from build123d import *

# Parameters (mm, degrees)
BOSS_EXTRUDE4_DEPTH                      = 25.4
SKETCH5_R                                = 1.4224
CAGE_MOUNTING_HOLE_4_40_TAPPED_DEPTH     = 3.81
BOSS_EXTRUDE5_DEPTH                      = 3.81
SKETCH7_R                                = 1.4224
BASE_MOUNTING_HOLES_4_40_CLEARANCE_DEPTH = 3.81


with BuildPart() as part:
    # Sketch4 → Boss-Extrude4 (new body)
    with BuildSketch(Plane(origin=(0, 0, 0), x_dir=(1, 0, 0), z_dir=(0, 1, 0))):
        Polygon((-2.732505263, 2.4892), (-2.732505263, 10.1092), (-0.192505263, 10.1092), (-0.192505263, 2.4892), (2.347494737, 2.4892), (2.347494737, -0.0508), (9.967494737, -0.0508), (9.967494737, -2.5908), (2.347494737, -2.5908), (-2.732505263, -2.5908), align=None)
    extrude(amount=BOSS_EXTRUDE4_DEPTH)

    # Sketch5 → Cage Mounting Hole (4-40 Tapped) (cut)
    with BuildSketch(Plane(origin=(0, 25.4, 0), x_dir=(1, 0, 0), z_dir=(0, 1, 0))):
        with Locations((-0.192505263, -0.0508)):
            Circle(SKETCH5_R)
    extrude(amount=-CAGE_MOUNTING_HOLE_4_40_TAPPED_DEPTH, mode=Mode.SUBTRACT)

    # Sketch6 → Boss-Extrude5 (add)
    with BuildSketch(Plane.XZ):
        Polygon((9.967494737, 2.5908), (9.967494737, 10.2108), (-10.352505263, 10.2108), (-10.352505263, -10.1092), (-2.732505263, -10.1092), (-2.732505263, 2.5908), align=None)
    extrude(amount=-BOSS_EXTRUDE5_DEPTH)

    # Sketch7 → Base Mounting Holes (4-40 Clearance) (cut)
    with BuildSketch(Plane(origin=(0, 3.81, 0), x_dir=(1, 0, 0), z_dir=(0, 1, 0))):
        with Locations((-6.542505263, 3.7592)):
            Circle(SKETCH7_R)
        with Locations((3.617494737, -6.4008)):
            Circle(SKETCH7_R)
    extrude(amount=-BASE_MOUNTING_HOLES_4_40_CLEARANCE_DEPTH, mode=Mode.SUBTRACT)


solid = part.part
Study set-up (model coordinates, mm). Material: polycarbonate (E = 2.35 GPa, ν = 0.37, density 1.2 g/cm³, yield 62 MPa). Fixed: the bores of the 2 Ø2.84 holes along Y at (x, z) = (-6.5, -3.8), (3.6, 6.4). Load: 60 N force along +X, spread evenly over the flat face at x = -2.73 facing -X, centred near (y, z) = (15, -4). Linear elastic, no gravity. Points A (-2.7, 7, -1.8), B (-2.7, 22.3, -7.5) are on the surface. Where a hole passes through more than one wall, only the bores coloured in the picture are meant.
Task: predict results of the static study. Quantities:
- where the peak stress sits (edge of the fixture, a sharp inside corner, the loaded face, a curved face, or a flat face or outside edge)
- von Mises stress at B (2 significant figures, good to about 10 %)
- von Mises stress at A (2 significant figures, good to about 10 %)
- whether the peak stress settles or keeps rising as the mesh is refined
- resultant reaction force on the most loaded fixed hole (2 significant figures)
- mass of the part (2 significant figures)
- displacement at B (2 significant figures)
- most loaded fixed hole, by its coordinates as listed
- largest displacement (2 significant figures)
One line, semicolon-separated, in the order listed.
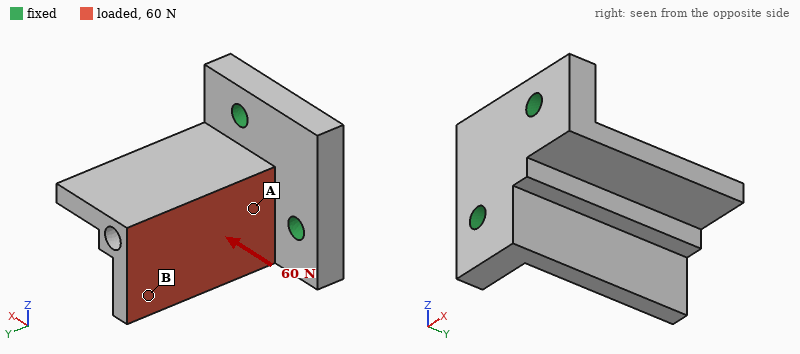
edge of the fixture; 1.7 MPa; 5.9 MPa; keeps rising; 60 N; 3.0 g; 0.33 mm; (-6.5, -3.8); 0.42 mm
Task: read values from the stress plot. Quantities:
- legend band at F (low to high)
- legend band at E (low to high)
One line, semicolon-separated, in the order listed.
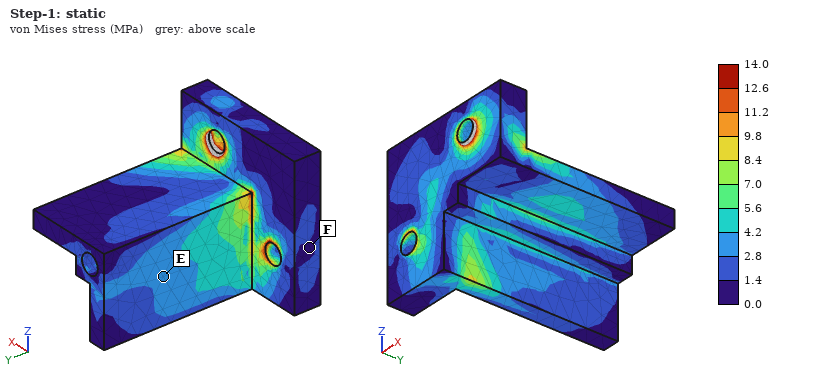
0.0 to 1.4 MPa; 2.8 to 4.2 MPa
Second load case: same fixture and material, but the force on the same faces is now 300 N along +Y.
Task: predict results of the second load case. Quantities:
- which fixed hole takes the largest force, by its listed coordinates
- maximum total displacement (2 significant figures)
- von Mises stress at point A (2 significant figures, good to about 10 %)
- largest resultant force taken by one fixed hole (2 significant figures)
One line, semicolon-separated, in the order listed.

(-6.5, -3.8); 0.35 mm; 14 MPa; 260 N
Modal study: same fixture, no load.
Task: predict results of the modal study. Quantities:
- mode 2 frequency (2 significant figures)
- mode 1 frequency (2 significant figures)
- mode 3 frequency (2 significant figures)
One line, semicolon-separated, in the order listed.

2900 Hz; 1900 Hz; 3700 Hz
